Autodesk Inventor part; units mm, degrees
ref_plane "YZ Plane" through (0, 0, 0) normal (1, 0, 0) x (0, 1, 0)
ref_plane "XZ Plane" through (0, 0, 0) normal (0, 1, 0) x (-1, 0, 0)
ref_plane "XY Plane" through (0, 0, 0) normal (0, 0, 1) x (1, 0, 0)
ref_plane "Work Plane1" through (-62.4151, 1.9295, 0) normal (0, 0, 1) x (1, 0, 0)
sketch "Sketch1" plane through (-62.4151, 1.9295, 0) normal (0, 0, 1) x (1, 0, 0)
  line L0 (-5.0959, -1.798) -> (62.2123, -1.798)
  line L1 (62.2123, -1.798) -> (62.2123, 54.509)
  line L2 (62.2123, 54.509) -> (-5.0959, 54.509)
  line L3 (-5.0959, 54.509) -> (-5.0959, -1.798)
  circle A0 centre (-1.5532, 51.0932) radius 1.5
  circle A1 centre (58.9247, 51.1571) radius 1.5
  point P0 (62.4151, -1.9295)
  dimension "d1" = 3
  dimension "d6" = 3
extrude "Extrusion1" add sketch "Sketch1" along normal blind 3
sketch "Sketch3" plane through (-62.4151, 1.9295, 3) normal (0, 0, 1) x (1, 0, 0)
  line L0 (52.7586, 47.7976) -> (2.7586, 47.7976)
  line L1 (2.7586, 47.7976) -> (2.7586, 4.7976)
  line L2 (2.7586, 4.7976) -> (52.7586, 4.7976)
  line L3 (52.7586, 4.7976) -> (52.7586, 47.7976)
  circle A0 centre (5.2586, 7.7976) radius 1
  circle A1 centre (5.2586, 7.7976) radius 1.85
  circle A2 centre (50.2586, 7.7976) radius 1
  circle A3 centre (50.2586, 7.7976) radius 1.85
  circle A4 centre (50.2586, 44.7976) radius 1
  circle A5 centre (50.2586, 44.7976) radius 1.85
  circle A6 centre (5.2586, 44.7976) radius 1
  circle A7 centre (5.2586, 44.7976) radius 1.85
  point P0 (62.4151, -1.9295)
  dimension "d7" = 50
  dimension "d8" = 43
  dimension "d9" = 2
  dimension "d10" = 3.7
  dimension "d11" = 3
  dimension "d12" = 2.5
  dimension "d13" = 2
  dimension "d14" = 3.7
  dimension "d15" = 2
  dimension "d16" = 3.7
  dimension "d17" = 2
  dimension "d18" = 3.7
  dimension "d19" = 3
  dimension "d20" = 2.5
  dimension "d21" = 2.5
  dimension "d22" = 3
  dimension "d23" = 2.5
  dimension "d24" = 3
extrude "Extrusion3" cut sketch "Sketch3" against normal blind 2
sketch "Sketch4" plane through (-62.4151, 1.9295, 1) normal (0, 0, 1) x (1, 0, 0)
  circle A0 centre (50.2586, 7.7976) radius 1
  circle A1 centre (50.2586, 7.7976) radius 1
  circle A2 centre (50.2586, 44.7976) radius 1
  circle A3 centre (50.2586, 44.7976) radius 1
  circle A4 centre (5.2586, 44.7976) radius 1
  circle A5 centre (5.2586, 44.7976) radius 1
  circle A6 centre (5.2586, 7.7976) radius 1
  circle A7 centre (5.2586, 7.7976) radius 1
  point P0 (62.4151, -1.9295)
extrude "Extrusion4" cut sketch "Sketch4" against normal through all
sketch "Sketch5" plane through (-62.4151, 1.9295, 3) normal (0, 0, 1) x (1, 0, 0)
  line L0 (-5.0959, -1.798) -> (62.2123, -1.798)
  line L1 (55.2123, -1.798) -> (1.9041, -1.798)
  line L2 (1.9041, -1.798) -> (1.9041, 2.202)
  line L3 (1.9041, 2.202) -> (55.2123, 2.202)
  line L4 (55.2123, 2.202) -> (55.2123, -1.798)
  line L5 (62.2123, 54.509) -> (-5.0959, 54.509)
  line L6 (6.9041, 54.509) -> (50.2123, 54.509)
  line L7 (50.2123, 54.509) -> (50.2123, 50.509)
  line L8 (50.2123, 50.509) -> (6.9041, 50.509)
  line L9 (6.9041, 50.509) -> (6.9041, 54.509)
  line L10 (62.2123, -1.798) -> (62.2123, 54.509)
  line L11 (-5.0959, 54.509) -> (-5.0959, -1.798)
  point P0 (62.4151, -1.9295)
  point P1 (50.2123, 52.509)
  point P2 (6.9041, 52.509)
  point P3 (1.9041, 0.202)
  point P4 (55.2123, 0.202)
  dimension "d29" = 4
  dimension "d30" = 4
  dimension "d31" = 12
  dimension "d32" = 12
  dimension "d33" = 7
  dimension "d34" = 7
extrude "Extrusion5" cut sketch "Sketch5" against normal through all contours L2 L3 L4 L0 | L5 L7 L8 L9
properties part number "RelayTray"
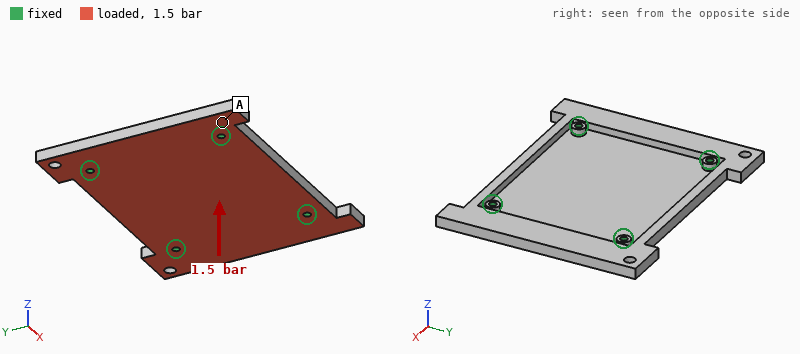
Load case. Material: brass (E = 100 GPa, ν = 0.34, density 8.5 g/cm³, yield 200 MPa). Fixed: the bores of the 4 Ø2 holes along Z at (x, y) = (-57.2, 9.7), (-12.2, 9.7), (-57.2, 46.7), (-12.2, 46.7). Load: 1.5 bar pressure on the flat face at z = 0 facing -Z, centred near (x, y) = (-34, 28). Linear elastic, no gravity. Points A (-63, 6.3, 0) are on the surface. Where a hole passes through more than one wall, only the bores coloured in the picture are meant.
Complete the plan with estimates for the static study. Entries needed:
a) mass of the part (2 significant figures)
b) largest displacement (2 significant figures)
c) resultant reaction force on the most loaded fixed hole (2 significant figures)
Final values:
50 g
0.17 mm
130 N
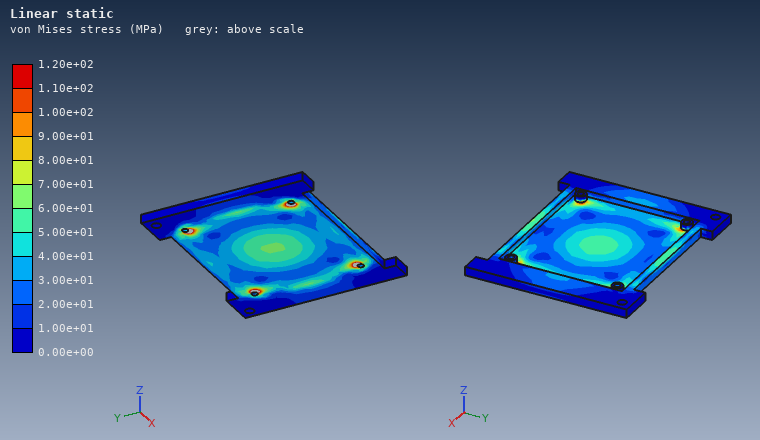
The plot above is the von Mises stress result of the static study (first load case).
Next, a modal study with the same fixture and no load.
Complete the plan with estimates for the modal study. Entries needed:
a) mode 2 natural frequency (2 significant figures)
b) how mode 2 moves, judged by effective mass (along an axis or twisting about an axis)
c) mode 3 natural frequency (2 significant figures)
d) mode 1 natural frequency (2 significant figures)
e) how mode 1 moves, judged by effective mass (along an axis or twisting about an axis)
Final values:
3000 Hz
along Z
3300 Hz
2000 Hz
along Z
